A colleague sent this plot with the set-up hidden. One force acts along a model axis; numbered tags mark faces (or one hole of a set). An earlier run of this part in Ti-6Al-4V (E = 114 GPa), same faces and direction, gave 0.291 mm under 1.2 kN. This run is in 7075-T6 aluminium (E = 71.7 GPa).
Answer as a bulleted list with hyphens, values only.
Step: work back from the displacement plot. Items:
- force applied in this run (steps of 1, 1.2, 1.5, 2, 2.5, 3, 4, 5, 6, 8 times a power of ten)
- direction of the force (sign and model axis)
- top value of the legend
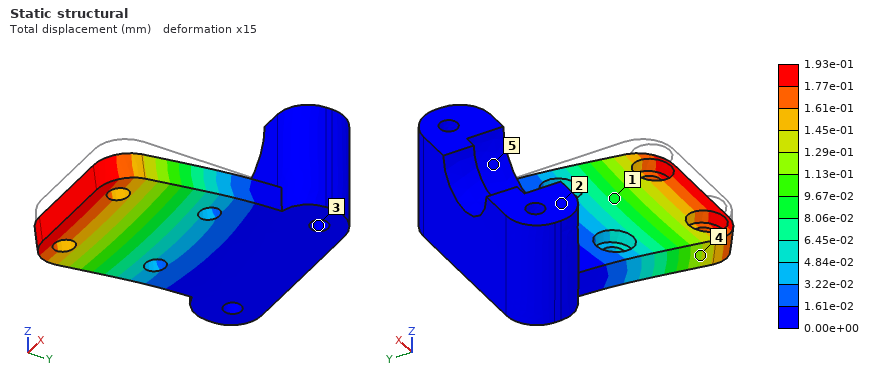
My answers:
- 500 N
- -Z
- 1.93e-01 mm
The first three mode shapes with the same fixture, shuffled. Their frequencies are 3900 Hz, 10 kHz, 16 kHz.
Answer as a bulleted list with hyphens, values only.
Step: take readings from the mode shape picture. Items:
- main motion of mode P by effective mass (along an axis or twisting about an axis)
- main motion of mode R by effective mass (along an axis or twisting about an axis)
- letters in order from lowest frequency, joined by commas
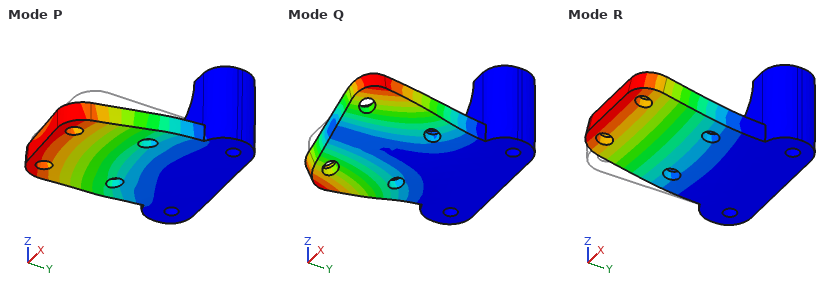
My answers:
- along X
- along Z
- R, Q, P
